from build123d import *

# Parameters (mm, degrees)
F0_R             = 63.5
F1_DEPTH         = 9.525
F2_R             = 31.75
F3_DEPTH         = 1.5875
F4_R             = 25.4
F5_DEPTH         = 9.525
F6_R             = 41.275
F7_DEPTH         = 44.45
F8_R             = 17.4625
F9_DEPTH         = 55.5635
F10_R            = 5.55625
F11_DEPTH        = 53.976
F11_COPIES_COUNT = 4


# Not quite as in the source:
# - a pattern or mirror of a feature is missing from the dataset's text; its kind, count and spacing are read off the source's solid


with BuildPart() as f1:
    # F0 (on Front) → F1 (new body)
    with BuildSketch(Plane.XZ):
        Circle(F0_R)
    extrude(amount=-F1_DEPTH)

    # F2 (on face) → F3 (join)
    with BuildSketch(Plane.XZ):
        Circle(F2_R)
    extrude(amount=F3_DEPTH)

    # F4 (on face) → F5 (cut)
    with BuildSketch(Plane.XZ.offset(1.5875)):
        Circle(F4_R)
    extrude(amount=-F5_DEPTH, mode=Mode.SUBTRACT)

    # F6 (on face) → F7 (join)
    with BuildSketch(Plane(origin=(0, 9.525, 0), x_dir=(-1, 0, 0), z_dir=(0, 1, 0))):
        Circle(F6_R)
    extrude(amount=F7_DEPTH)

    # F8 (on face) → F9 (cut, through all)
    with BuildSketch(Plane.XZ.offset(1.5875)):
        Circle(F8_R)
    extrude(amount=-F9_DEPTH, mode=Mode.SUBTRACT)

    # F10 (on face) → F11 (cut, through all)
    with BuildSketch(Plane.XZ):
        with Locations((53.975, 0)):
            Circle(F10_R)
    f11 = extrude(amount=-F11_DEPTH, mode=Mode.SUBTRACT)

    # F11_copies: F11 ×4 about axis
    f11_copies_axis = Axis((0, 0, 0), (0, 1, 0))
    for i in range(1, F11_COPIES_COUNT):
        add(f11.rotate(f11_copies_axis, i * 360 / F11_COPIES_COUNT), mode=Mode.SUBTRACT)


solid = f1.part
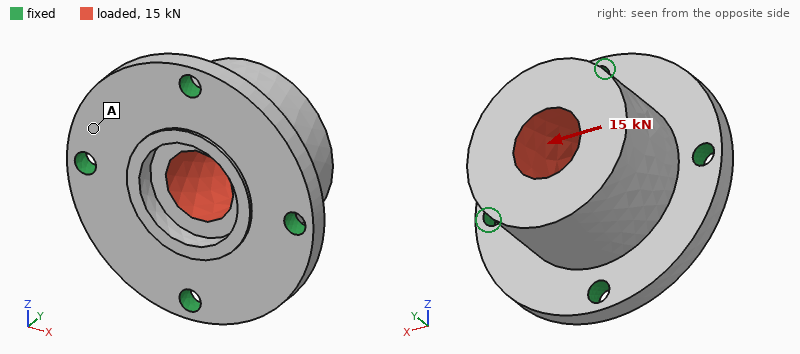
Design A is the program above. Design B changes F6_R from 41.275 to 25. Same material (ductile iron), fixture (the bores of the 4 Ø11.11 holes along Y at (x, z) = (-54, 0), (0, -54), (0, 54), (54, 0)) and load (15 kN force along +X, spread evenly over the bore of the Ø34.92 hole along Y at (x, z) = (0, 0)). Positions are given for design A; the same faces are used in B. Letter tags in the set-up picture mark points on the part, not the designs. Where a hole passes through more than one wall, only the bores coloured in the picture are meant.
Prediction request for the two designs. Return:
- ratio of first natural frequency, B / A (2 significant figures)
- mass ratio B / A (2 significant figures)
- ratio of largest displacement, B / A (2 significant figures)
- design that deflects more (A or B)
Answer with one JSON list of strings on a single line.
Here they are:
["0.79", "0.49", "7.1", "B"]
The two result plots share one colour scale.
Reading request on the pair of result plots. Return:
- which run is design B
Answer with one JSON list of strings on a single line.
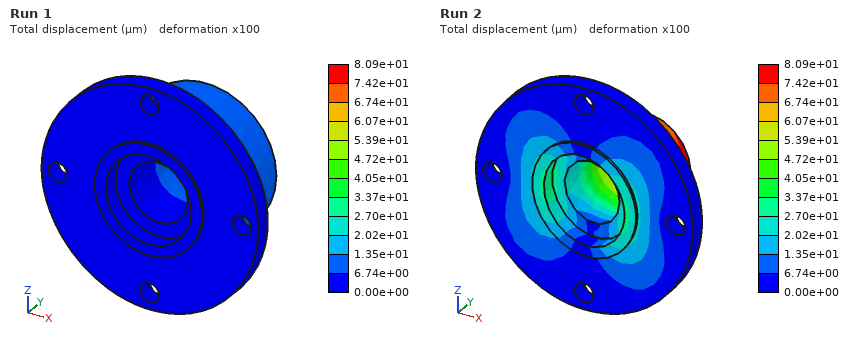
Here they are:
["Run 2"]
